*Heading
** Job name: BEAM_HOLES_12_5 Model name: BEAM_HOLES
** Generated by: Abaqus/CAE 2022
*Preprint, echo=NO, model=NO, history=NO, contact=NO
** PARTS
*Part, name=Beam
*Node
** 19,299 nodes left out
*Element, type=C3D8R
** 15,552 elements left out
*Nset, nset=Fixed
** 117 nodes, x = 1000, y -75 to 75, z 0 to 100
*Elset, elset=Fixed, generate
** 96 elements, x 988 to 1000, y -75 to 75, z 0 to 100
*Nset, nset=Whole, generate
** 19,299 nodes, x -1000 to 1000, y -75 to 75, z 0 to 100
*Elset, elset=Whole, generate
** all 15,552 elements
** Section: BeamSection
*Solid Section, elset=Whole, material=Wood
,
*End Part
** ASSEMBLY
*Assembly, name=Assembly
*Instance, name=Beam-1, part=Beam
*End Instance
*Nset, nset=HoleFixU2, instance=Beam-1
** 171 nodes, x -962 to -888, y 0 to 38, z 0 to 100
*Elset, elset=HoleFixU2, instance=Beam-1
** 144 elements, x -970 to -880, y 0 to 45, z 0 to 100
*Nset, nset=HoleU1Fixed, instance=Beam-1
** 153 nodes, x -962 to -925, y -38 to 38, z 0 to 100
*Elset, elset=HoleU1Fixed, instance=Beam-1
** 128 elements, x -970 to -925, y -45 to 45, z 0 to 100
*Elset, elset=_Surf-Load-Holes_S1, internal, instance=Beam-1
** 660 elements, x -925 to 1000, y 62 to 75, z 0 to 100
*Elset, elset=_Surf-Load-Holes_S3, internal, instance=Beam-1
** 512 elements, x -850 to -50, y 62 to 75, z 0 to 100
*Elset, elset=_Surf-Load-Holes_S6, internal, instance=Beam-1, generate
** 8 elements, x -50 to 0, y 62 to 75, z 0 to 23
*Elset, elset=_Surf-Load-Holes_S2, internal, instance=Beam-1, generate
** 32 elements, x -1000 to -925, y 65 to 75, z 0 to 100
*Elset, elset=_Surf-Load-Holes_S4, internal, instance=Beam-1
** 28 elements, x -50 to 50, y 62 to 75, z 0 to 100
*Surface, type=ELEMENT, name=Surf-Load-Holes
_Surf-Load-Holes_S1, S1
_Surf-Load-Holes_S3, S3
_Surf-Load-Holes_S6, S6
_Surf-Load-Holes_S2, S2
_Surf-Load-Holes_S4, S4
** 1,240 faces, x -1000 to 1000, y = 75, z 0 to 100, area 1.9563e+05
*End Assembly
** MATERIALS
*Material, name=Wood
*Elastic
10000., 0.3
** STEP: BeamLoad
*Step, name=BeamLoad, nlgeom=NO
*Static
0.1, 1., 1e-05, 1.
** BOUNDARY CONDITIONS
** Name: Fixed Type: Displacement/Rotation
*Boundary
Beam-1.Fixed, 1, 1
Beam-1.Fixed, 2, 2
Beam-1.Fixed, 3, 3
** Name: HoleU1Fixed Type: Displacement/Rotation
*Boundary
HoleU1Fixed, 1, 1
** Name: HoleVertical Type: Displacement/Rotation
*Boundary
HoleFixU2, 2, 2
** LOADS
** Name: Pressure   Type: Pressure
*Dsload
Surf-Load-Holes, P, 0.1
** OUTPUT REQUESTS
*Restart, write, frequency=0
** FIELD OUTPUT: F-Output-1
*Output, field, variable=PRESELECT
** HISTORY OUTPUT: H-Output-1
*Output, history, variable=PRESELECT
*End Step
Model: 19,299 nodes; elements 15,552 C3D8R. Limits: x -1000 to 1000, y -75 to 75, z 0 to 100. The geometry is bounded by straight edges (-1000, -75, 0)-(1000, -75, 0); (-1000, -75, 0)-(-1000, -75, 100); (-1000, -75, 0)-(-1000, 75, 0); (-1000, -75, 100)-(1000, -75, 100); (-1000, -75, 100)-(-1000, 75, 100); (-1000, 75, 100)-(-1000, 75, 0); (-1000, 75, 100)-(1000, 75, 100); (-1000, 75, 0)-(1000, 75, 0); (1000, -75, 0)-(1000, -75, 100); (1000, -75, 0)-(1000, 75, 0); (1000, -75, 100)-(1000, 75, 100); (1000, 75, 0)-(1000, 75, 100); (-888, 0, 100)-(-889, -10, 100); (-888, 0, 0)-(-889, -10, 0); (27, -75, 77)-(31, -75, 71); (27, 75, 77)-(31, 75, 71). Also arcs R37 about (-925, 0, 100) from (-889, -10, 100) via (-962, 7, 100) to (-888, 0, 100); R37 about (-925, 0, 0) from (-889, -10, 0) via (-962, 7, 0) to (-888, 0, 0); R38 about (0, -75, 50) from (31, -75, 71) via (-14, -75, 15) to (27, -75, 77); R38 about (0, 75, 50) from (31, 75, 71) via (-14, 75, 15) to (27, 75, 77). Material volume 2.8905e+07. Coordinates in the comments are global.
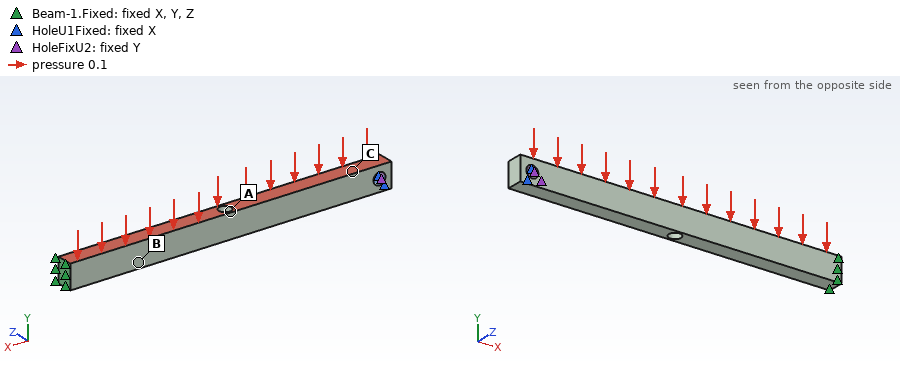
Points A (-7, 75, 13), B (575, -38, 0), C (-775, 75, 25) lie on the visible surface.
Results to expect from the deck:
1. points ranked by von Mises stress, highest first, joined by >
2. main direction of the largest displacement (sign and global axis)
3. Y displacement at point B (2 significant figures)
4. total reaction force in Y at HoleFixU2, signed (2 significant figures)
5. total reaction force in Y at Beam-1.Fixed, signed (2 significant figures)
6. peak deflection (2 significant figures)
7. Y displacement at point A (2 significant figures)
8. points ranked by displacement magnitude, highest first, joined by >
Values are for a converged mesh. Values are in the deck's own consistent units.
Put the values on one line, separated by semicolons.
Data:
A > C > B; -Y; -0.72; 9900; 9600; 1.7; -1.7; A > B > C
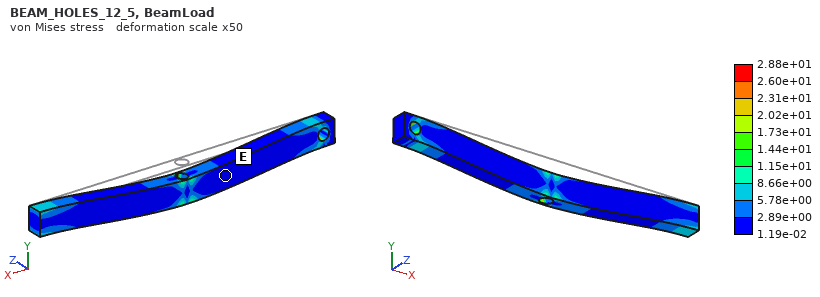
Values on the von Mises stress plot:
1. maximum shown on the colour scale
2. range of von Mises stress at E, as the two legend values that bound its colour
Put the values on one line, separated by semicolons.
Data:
2.88e+01; 1.19e-02 to 2.89e+00
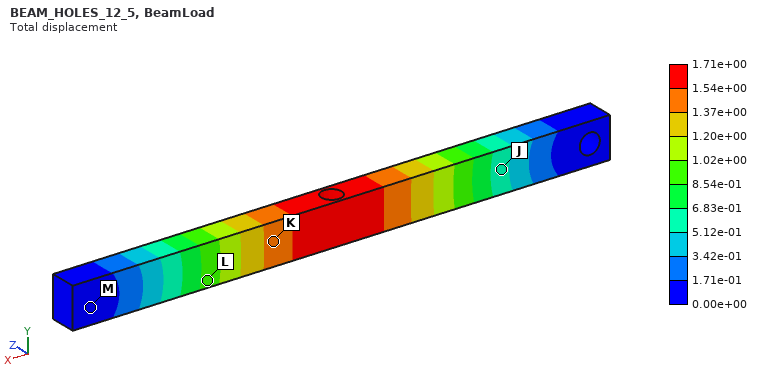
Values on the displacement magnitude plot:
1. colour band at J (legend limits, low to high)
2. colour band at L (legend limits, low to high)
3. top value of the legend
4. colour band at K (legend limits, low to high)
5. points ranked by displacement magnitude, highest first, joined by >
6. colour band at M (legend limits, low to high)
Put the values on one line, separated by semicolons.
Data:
5.12e-01 to 6.83e-01; 8.54e-01 to 1.02e+00; 1.71e+00; 1.37e+00 to 1.54e+00; K > L > J > M; 0.00e+00 to 1.71e-01
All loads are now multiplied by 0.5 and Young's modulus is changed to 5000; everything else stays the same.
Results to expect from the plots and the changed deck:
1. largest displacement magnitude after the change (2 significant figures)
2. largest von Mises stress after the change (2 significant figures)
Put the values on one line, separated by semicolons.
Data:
1.7; 14
